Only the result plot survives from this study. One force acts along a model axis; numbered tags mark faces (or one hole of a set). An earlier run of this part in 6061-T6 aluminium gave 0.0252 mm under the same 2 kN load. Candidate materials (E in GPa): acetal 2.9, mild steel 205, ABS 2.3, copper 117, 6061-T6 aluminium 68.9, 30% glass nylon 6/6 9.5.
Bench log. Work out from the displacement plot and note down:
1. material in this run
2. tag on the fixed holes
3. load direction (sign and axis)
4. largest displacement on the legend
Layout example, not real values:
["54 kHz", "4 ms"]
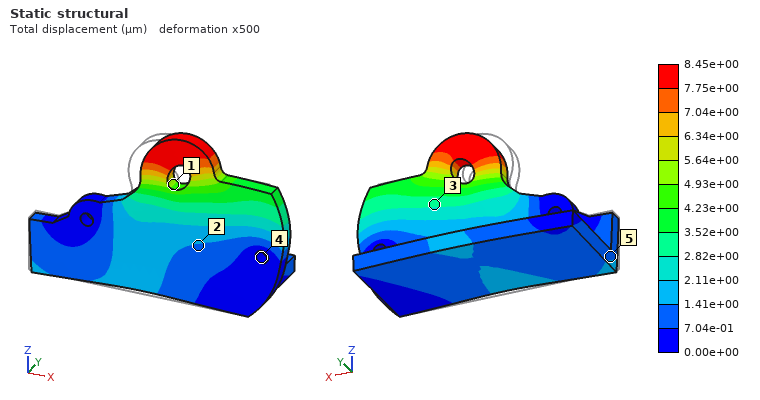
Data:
["mild steel", "4", "+X", "8.45e+00 µm"]
